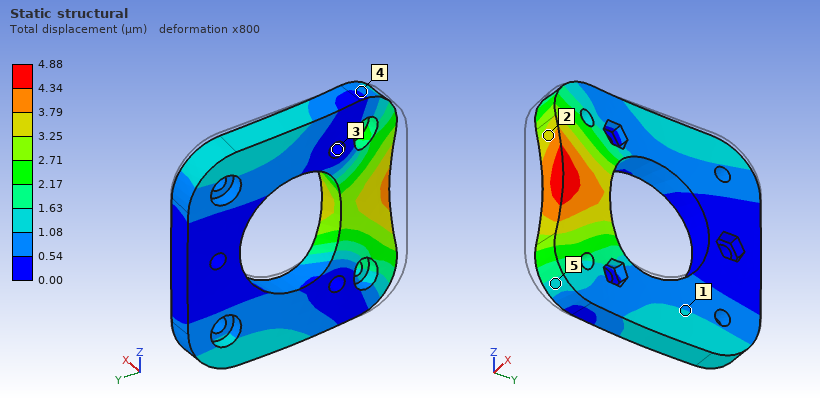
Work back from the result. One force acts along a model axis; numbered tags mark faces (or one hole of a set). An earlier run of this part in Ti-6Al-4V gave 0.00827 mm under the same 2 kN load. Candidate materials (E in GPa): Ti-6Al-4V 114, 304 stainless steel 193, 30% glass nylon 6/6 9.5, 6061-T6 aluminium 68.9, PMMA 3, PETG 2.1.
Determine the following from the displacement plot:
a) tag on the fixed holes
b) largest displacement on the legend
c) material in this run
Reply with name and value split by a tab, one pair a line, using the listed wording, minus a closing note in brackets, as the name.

tag on the fixed holes	3
largest displacement on the legend	4.88 µm
material in this run	304 stainless steel
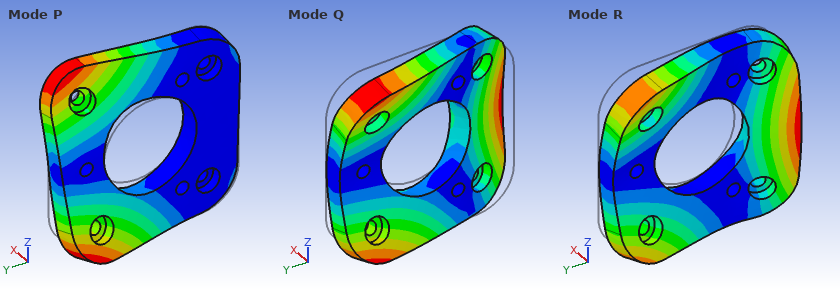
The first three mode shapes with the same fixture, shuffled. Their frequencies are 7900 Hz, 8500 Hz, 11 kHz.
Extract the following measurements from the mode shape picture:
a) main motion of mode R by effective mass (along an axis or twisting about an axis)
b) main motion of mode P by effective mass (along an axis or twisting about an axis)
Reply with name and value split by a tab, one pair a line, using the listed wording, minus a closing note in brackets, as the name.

main motion of mode R by effective mass	along X
main motion of mode P by effective mass	twisting about Y
